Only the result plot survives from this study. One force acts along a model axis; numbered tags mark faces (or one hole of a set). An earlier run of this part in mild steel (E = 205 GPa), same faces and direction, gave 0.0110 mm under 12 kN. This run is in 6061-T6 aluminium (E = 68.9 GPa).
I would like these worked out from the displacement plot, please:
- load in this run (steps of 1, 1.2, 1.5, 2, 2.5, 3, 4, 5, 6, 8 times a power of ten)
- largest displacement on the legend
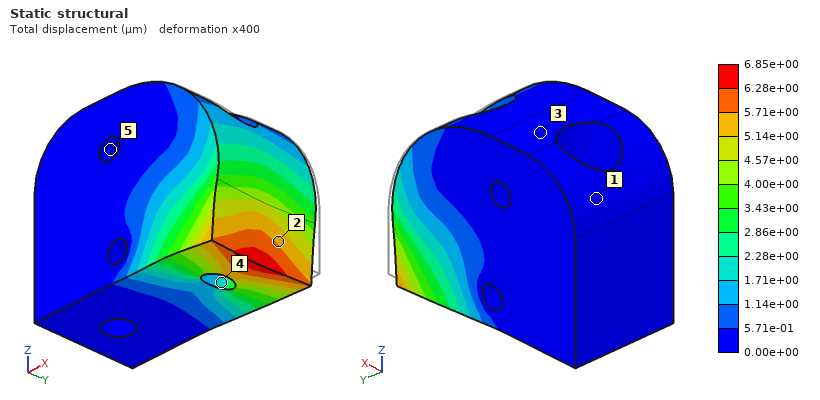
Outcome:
2.5 kN
6.85e+00 µm
